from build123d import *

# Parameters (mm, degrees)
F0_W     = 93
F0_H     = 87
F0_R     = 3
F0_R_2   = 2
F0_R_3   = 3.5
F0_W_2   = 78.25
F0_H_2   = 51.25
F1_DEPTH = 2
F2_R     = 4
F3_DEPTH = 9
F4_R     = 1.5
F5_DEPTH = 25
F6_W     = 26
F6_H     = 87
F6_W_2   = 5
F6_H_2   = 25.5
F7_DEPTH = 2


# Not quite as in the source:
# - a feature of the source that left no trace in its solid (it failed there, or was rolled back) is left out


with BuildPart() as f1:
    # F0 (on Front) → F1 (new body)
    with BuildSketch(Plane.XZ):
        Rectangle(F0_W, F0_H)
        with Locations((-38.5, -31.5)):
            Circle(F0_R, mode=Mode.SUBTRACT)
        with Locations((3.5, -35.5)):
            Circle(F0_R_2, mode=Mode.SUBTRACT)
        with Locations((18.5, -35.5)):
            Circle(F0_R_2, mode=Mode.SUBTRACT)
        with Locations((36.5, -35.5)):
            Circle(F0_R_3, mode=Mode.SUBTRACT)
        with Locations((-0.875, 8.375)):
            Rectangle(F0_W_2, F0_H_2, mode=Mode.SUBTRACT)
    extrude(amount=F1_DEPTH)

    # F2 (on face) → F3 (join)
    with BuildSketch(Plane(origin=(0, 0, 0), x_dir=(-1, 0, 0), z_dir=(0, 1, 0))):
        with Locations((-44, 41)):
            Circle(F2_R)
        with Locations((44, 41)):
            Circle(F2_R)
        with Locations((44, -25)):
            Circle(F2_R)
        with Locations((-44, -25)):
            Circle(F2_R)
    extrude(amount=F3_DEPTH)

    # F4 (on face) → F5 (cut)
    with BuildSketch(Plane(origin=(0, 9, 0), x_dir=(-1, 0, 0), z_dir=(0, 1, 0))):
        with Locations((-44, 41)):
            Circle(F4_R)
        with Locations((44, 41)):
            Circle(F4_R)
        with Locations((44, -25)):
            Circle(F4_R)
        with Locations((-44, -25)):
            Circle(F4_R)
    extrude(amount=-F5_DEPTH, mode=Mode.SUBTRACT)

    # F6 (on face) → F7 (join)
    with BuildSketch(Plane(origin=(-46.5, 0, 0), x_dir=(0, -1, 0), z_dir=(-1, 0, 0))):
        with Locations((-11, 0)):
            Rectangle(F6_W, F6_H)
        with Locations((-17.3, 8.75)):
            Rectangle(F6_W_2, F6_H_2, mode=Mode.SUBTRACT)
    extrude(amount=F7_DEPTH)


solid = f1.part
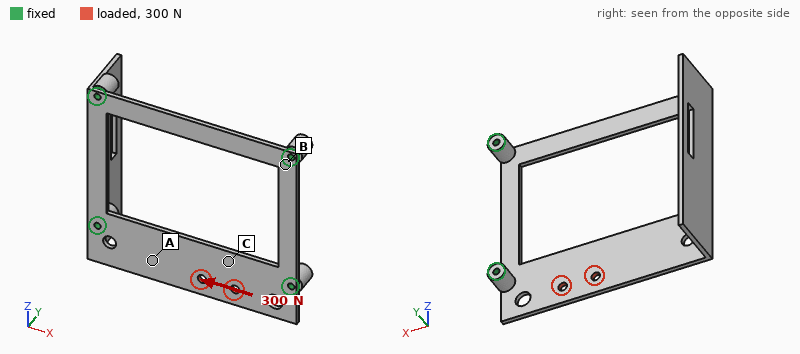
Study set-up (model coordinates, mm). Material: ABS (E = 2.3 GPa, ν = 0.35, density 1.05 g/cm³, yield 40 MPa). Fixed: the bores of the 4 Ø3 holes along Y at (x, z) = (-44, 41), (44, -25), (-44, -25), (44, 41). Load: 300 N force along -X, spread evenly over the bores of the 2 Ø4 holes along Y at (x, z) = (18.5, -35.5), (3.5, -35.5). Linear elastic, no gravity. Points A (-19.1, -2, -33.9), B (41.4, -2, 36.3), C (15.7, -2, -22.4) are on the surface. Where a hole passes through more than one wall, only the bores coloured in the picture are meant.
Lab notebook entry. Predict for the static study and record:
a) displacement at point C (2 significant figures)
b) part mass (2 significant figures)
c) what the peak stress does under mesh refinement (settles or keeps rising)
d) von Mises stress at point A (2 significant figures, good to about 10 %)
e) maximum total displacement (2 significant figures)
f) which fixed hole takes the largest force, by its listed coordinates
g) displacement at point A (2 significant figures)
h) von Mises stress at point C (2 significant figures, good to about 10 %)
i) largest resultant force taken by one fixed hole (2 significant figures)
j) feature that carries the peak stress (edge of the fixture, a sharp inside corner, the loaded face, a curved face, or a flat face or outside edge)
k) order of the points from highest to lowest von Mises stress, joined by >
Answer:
0.060 mm
14 g
keeps rising
3.0 MPa
0.11 mm
(44, -25)
0.053 mm
2.1 MPa
170 N
edge of the fixture
A > C > B
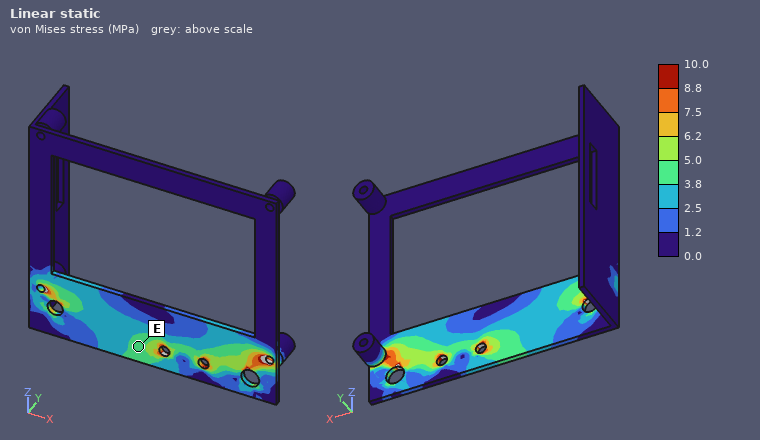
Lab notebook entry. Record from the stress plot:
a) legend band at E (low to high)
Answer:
3.8 to 5.0 MPa
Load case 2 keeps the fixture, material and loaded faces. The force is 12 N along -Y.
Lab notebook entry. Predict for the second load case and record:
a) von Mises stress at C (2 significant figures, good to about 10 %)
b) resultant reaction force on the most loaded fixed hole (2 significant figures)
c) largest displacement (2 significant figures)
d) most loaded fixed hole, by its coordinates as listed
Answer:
3.4 MPa
8.8 N
1.3 mm
(44, -25)
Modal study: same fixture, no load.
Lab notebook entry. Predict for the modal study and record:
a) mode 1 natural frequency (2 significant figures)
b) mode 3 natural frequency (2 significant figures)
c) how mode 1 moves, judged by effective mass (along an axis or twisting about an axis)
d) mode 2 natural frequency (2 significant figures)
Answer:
380 Hz
800 Hz
along Y
440 Hz
